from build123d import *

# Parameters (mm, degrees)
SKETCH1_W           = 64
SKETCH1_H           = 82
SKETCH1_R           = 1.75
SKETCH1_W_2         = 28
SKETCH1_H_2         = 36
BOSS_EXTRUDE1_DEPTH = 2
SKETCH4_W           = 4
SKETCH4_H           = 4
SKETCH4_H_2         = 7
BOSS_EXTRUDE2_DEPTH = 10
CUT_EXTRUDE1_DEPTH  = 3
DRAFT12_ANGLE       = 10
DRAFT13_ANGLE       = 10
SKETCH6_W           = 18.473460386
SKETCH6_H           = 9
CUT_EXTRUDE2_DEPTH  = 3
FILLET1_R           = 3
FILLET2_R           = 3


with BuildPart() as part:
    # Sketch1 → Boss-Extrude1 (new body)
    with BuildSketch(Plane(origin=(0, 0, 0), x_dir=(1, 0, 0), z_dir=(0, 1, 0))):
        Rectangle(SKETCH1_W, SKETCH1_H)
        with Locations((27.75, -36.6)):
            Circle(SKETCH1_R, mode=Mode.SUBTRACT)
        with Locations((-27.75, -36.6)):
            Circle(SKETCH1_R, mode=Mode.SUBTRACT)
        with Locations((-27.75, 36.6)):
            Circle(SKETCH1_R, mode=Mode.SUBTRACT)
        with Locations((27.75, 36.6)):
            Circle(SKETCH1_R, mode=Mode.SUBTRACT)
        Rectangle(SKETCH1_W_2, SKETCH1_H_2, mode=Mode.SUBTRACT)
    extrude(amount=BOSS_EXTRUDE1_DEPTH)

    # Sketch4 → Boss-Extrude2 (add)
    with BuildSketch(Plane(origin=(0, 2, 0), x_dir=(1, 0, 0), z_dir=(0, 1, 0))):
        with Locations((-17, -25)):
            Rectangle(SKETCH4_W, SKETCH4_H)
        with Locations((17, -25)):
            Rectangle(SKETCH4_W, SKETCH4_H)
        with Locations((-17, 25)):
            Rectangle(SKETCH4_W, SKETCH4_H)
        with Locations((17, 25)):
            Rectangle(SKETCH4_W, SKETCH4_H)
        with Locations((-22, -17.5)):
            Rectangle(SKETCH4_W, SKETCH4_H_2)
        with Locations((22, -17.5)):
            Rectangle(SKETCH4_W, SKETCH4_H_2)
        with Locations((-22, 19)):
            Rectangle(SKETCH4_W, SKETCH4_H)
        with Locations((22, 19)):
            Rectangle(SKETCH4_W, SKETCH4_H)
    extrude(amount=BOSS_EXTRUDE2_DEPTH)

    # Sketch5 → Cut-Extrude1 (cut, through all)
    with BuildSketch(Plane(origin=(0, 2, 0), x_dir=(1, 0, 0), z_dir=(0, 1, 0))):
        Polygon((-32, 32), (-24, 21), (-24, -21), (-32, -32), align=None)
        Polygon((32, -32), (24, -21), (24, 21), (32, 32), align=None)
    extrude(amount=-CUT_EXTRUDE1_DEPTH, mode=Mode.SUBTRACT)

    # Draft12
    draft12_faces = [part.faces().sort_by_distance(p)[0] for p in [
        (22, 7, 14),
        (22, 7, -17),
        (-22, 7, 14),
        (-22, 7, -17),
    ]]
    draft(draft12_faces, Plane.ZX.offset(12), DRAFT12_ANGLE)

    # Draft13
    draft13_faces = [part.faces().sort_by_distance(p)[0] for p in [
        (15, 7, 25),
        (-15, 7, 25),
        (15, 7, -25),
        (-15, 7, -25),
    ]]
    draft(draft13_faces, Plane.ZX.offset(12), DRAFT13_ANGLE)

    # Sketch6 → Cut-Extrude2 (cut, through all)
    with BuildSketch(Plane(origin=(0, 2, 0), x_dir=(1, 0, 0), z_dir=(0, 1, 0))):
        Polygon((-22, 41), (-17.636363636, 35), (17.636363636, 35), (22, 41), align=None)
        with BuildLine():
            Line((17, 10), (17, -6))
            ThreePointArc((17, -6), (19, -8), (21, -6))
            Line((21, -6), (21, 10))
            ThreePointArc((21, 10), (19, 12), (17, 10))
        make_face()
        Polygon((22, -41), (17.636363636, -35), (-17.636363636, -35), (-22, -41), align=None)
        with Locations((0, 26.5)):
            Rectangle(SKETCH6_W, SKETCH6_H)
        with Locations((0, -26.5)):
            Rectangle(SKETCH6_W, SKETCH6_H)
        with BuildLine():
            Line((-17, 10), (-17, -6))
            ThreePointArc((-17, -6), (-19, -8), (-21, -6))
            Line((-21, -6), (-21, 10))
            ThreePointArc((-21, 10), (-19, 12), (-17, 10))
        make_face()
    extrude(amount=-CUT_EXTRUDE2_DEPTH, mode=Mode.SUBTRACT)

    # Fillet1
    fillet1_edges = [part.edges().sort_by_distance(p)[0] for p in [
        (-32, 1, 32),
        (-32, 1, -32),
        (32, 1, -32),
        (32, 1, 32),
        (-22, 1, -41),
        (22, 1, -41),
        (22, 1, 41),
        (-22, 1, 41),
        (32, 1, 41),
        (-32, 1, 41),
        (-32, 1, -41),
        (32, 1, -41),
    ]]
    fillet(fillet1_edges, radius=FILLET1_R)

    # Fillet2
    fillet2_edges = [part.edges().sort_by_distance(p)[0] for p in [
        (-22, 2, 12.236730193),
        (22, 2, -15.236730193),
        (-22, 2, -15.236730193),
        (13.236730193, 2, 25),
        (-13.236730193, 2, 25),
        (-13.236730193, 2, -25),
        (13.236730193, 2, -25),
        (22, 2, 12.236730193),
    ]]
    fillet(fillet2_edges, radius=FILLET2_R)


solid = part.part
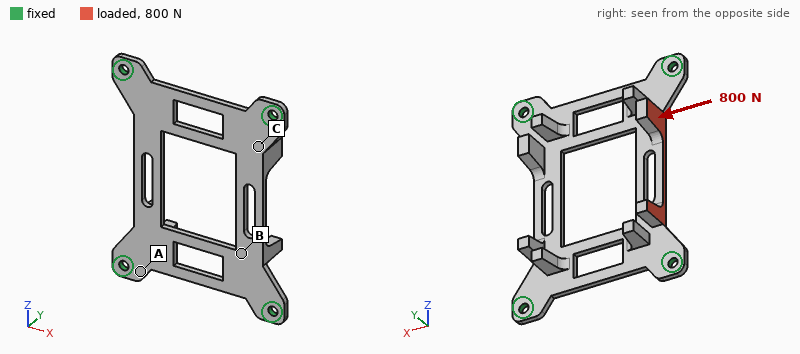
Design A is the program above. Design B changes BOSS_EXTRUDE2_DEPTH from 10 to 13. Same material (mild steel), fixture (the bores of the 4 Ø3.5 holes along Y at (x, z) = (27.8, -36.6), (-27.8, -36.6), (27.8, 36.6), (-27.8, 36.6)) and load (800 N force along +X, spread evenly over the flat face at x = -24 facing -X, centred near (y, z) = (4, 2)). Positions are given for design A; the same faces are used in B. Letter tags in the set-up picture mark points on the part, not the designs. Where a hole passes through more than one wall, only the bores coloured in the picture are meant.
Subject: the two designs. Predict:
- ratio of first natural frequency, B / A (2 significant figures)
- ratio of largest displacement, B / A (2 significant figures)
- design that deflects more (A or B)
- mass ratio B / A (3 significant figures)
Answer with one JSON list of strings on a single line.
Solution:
["0.95", "1.6", "B", "1.07"]
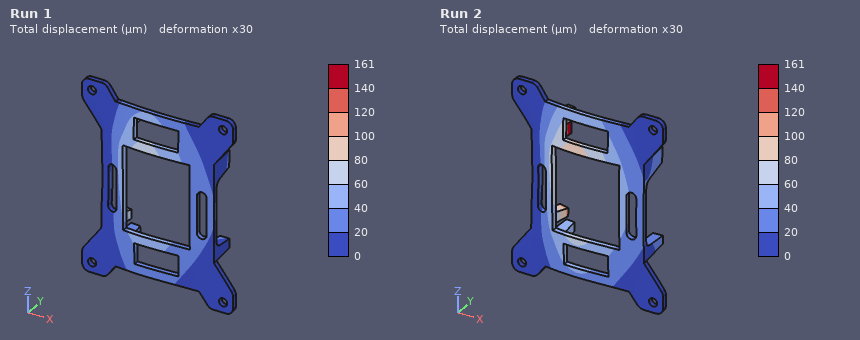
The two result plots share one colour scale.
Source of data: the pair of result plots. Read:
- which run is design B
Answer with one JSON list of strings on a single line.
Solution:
["Run 2"]
